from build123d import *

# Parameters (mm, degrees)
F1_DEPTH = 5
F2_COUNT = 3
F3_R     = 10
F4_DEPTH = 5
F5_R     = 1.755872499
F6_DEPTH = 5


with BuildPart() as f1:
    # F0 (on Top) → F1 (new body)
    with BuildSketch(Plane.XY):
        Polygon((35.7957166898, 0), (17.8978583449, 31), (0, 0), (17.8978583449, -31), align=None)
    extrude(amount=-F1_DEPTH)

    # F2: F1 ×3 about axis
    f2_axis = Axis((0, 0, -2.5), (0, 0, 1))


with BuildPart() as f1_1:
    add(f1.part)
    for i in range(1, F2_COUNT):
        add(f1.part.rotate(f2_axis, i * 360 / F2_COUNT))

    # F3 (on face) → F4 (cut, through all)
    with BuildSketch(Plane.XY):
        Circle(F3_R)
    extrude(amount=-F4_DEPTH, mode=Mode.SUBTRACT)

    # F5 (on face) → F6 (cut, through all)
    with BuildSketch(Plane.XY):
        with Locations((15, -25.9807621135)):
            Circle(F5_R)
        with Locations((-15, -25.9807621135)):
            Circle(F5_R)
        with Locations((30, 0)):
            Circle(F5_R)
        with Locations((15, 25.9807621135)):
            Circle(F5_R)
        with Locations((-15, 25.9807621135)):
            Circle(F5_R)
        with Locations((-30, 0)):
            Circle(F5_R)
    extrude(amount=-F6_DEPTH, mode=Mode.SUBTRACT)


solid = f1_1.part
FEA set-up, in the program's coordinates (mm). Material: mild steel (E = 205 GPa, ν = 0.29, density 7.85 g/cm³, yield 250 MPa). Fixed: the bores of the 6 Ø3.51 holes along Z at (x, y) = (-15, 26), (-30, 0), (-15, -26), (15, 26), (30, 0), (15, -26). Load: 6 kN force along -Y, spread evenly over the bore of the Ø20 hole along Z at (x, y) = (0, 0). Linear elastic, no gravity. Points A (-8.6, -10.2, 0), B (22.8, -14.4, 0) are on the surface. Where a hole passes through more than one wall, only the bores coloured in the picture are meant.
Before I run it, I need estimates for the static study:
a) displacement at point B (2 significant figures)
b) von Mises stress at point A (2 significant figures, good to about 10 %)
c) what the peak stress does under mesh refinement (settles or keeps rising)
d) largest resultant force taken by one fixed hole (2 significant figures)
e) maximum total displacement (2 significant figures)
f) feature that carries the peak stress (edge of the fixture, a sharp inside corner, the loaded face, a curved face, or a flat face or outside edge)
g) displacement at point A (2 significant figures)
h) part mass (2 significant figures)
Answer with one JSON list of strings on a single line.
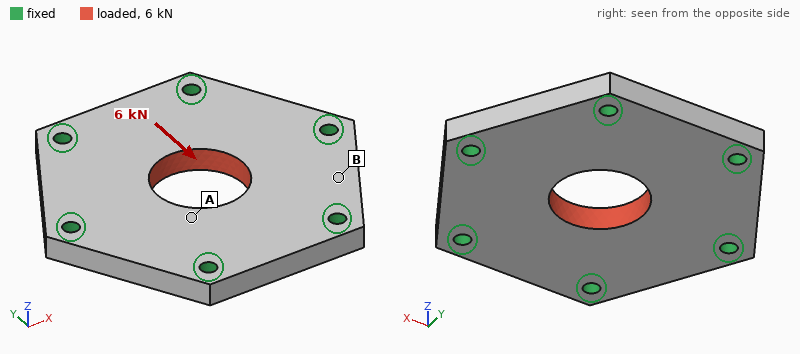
["0.81 µm", "20 MPa", "keeps rising", "1.3 kN", "2.3 µm", "edge of the fixture", "1.8 µm", "120 g"]
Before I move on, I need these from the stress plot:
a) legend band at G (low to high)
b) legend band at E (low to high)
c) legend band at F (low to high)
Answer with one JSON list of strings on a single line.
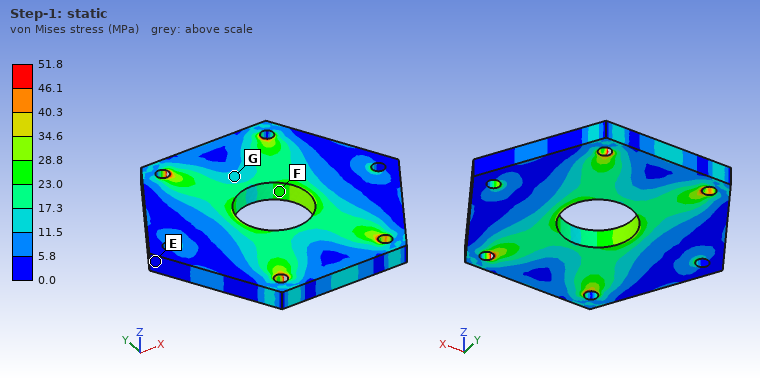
["11.5 to 17.3 MPa", "0.0 to 5.8 MPa", "23.0 to 28.8 MPa"]
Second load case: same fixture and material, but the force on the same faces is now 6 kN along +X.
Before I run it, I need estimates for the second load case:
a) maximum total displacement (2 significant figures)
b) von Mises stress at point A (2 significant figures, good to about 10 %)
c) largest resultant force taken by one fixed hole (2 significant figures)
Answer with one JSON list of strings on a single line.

["2.3 µm", "16 MPa", "1.5 kN"]
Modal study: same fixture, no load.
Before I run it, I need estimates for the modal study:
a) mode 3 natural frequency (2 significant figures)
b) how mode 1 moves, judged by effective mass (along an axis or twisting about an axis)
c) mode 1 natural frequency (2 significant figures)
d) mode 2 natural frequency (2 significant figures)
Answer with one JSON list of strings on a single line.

["19 kHz", "along Z", "12 kHz", "19 kHz"]
